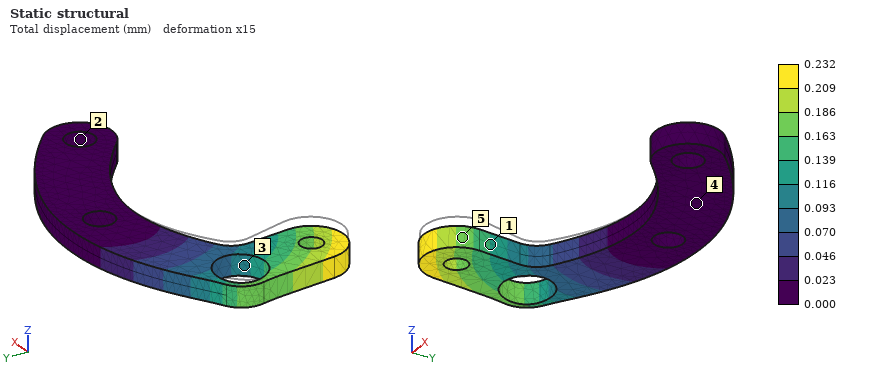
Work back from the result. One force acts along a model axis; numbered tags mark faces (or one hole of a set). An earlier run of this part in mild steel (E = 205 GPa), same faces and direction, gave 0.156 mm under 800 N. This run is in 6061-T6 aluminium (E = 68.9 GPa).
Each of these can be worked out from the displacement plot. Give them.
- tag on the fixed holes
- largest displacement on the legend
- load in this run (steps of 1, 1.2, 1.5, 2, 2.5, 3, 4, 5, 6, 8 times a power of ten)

2
0.232 mm
400 N
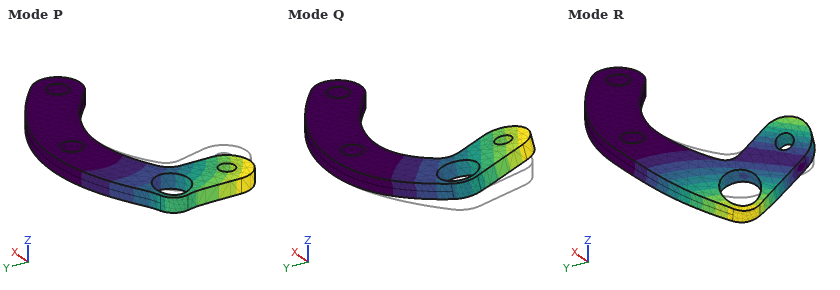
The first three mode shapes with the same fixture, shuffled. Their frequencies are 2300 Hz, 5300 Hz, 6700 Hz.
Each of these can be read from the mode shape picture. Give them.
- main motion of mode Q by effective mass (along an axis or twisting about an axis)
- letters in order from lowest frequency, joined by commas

along Z
Q, P, R
